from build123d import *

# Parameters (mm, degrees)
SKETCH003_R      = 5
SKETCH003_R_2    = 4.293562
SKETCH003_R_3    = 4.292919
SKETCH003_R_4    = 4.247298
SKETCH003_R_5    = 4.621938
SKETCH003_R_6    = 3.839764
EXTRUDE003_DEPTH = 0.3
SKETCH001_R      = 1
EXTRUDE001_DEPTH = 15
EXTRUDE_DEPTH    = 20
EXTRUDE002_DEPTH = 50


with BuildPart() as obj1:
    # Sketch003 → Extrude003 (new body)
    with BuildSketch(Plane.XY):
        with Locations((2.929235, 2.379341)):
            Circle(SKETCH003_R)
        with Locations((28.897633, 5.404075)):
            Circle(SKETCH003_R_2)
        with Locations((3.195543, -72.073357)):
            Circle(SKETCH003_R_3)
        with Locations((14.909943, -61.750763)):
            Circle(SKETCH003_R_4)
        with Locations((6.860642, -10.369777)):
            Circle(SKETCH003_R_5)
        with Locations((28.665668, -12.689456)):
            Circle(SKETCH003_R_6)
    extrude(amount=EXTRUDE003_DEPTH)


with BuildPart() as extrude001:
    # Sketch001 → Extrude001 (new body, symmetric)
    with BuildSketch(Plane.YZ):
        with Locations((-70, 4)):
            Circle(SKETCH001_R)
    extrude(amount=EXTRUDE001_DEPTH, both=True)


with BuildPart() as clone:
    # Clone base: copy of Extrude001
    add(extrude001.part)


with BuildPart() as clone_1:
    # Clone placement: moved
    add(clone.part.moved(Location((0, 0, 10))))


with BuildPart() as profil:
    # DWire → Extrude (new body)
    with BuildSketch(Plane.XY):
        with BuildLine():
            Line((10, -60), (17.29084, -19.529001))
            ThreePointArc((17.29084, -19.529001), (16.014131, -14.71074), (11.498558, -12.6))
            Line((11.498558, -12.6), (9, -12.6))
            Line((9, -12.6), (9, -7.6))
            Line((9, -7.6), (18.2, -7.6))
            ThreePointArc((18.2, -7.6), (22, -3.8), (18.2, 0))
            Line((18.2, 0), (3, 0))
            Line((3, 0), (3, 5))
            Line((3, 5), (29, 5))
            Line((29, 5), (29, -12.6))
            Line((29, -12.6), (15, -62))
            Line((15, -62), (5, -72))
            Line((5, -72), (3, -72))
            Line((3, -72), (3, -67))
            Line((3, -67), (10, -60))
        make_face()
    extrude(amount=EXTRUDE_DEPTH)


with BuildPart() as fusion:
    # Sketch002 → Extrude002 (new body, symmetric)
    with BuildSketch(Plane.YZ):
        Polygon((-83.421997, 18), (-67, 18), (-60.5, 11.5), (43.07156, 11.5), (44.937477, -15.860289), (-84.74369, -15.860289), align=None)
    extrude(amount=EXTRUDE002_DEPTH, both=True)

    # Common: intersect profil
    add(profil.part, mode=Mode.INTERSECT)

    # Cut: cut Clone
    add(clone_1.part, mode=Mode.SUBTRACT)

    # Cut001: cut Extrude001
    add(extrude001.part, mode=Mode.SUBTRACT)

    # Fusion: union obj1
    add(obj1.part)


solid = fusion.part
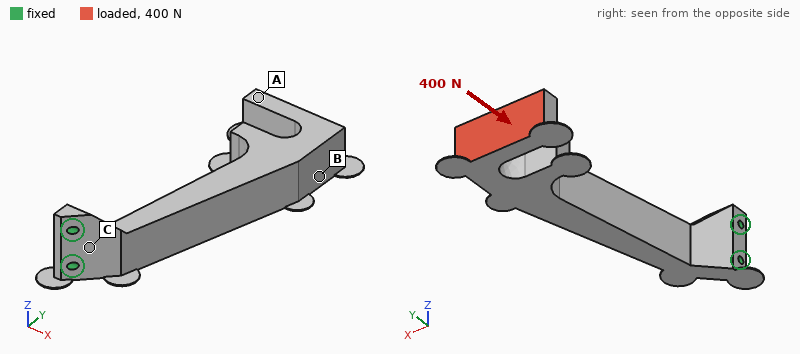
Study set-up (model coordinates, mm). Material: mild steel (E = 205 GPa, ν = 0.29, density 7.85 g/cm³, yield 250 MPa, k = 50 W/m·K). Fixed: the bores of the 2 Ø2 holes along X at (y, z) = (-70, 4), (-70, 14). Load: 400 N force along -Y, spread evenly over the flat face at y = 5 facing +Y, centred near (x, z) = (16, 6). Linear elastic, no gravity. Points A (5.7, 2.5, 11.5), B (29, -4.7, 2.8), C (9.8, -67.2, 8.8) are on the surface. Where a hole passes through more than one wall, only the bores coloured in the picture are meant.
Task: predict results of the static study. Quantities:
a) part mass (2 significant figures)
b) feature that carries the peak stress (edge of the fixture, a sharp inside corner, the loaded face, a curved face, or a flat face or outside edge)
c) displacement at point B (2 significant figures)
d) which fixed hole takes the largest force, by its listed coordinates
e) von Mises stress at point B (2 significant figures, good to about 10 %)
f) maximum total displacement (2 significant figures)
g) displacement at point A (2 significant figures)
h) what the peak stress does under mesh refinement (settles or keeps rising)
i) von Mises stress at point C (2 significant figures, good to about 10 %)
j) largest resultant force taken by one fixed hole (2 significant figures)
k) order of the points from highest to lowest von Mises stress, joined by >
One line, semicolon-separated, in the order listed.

70 g; edge of the fixture; 0.092 mm; (-70, 4); 31 MPa; 0.10 mm; 0.095 mm; keeps rising; 46 MPa; 320 N; C > B > A
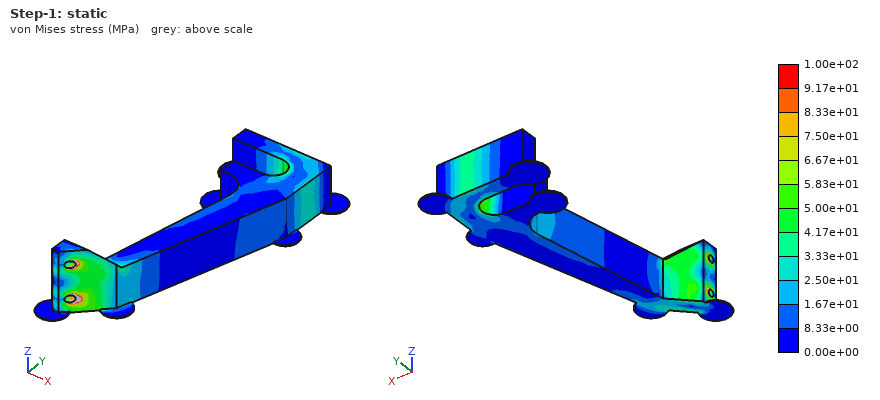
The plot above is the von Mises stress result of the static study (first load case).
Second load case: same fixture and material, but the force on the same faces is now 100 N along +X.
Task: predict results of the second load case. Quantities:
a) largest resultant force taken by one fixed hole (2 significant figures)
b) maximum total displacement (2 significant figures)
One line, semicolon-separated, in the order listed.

60 N; 0.43 mm
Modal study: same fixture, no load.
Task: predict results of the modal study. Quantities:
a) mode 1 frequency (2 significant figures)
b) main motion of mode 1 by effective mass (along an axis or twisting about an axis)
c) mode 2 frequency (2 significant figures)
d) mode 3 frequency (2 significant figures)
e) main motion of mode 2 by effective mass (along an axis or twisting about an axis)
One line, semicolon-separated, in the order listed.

480 Hz; along X; 930 Hz; 3500 Hz; along Z
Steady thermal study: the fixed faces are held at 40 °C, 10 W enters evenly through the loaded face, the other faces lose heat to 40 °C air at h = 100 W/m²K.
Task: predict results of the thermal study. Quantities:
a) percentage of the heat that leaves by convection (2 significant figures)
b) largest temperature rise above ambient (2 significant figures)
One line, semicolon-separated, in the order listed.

90 %; 56 K
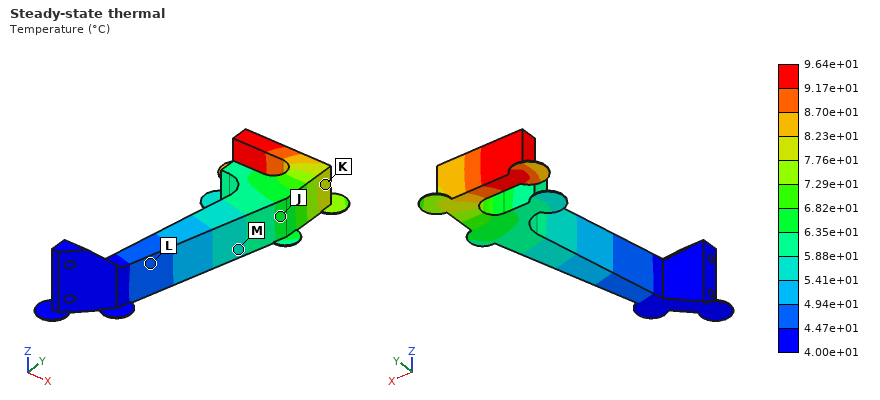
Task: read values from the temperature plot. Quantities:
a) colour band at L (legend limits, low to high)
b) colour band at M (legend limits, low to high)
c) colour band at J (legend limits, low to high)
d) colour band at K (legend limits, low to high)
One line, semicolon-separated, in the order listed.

4.47e+01 to 4.94e+01 °C; 5.41e+01 to 5.88e+01 °C; 6.35e+01 to 6.82e+01 °C; 7.76e+01 to 8.23e+01 °C
